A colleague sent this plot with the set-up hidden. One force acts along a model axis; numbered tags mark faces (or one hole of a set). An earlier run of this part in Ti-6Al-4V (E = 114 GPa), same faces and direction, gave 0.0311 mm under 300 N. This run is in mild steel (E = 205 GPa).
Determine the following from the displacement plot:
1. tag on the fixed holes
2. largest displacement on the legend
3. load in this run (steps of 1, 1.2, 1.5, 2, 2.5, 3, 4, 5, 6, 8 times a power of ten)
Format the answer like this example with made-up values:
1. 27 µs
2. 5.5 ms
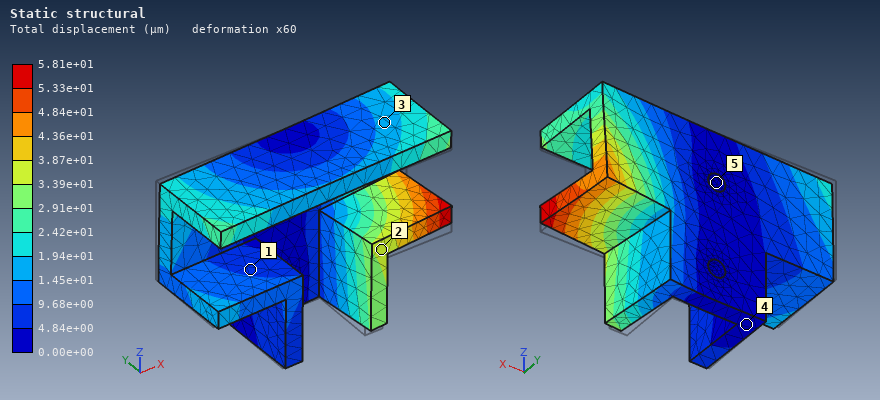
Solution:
1. 5
2. 5.81e+01 µm
3. 1 kN
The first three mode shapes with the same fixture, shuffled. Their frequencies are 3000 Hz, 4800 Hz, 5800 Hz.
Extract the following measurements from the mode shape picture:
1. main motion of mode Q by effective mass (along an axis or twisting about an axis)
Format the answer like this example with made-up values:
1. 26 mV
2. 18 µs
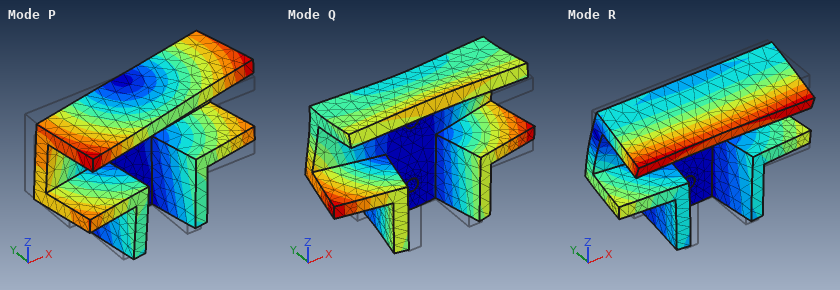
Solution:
1. along Y
